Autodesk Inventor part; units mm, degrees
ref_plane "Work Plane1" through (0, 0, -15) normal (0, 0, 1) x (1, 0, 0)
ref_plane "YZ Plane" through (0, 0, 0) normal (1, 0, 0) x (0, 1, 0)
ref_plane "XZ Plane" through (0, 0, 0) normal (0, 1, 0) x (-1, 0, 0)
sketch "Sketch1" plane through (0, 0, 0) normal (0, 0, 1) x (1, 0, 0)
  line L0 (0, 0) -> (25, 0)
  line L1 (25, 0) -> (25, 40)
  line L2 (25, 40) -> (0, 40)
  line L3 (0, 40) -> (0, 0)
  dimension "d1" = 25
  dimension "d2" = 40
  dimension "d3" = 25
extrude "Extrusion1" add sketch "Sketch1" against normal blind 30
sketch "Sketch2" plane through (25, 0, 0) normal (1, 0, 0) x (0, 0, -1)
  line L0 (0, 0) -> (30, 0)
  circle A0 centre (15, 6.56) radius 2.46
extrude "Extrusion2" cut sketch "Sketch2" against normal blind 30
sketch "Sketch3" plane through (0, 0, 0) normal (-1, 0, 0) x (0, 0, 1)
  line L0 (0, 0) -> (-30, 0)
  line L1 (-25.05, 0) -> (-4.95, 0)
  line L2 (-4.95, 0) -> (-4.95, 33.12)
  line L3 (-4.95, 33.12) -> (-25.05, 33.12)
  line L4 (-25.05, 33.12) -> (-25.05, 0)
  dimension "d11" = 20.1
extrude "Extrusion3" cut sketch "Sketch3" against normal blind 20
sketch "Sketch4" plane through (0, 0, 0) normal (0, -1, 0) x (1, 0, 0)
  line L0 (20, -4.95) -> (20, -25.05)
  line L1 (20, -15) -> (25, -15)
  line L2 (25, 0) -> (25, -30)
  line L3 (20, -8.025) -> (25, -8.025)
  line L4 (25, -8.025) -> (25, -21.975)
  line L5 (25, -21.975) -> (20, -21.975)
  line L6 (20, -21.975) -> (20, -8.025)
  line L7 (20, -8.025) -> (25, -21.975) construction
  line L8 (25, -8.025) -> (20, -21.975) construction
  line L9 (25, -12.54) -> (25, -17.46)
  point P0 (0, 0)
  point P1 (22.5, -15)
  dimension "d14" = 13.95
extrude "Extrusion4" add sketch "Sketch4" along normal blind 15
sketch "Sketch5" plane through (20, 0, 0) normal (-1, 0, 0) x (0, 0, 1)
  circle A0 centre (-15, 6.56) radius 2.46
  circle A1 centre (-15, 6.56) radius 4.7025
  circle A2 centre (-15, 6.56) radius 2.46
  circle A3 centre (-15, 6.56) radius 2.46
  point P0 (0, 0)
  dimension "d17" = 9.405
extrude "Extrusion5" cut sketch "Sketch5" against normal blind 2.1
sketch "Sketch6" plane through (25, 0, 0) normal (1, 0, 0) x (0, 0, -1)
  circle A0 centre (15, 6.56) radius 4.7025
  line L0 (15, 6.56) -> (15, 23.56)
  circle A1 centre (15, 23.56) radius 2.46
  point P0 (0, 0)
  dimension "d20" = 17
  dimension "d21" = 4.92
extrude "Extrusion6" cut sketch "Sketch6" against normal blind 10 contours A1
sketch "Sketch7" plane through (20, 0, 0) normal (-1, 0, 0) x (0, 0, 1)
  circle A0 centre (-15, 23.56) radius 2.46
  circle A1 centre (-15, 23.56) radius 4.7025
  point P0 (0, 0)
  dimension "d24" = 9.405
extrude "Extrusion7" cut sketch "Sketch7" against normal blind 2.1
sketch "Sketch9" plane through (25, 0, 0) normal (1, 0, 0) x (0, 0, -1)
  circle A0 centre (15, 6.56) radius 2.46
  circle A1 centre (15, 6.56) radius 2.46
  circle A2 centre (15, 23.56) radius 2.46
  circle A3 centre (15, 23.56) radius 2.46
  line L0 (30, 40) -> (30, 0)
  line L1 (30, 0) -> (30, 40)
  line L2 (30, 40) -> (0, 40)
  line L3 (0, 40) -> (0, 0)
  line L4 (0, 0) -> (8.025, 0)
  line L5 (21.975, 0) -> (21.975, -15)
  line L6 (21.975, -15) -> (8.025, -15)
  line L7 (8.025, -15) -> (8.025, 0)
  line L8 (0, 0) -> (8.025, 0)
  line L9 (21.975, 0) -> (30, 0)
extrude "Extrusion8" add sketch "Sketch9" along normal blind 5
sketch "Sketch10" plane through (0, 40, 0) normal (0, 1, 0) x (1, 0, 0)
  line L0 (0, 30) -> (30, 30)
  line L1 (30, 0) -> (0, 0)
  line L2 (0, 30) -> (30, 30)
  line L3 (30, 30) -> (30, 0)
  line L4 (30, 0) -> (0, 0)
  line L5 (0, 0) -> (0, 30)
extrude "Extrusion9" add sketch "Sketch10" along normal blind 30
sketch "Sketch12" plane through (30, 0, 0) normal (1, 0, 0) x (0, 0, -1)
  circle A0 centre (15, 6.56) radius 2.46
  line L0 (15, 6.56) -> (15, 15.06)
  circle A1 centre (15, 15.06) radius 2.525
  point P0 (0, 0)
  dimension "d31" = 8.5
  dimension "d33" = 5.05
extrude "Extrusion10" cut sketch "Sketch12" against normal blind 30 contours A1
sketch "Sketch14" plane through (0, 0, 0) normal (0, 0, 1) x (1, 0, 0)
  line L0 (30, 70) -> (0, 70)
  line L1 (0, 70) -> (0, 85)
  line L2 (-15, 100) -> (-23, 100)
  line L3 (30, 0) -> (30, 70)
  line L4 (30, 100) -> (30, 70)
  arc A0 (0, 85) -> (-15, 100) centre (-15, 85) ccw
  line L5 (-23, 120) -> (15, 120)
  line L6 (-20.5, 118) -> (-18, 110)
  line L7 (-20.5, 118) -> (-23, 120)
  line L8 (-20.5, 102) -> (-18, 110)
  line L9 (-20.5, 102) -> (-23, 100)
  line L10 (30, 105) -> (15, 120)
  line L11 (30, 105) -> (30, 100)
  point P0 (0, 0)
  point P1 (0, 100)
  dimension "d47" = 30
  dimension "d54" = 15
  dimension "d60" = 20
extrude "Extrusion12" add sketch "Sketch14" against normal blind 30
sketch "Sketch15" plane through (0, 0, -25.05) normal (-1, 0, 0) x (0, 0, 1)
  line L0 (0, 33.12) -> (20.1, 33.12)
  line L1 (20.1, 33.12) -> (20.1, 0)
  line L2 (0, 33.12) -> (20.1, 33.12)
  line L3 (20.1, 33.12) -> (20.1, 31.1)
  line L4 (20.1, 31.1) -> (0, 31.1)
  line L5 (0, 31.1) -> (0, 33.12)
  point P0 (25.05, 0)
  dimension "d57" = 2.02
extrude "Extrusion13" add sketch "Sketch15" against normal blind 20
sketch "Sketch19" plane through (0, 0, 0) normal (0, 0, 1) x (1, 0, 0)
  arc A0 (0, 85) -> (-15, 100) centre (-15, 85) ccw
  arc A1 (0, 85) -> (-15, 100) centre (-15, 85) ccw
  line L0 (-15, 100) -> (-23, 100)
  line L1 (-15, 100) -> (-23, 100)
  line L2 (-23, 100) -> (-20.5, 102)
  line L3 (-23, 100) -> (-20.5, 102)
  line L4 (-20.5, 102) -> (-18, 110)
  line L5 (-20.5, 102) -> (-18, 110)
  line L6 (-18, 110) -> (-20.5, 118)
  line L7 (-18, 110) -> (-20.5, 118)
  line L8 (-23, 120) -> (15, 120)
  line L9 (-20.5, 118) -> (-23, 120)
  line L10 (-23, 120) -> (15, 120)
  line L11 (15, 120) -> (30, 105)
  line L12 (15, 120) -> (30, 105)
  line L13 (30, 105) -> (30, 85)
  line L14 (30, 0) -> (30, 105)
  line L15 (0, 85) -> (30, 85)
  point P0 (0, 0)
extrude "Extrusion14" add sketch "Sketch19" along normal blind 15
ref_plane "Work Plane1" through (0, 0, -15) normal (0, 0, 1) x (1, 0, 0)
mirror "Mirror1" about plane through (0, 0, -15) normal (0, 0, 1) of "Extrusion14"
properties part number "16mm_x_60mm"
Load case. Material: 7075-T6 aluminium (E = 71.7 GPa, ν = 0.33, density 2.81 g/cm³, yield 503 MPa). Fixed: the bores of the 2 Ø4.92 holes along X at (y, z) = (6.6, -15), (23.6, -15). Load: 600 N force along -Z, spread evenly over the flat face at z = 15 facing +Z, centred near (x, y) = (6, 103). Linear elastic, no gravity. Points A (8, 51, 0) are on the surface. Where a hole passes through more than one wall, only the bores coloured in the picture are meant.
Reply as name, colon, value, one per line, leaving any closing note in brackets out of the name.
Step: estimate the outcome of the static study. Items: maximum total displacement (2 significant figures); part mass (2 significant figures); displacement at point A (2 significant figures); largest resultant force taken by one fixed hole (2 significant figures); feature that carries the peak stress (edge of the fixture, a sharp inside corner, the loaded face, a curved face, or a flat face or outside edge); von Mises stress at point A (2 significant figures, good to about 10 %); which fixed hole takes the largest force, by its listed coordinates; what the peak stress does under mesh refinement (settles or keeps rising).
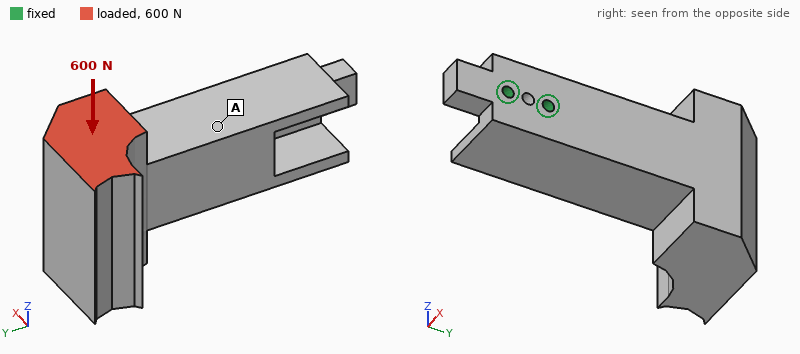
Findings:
maximum total displacement: 0.11 mm
part mass: 420 g
displacement at point A: 0.029 mm
largest resultant force taken by one fixed hole: 2.7 kN
feature that carries the peak stress: edge of the fixture
von Mises stress at point A: 6.9 MPa
which fixed hole takes the largest force, by its listed coordinates: (23.6, -15)
what the peak stress does under mesh refinement: keeps rising
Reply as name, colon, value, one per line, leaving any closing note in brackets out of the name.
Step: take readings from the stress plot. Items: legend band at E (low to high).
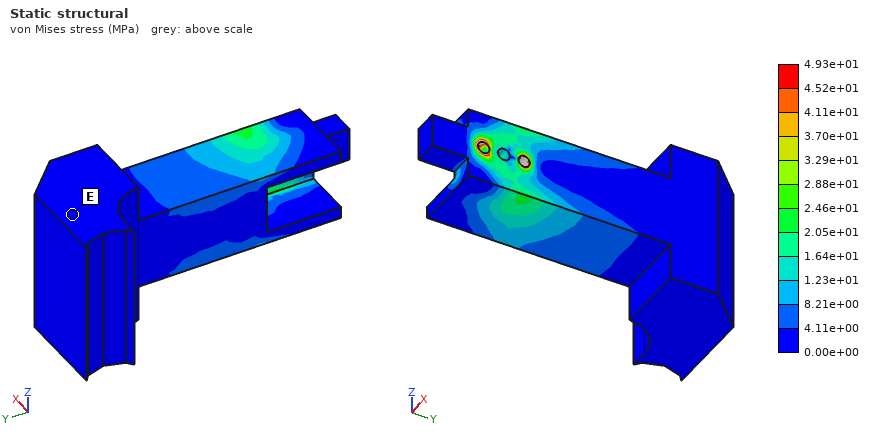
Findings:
legend band at E: 0.00e+00 to 4.11e+00 MPa
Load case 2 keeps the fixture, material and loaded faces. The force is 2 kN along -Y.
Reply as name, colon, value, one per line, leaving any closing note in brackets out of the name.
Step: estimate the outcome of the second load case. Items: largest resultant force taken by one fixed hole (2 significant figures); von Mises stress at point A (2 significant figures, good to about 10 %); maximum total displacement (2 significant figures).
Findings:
largest resultant force taken by one fixed hole: 3.2 kN
von Mises stress at point A: 16 MPa
maximum total displacement: 0.19 mm
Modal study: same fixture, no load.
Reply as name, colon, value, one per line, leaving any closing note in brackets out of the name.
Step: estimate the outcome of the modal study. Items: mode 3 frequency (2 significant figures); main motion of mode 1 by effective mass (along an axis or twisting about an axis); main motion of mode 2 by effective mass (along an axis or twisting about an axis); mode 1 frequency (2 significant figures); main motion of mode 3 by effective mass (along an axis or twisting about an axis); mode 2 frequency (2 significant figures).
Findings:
mode 3 frequency: 1800 Hz
main motion of mode 1 by effective mass: along X
main motion of mode 2 by effective mass: along Z
mode 1 frequency: 730 Hz
main motion of mode 3 by effective mass: twisting about Y
mode 2 frequency: 840 Hz
